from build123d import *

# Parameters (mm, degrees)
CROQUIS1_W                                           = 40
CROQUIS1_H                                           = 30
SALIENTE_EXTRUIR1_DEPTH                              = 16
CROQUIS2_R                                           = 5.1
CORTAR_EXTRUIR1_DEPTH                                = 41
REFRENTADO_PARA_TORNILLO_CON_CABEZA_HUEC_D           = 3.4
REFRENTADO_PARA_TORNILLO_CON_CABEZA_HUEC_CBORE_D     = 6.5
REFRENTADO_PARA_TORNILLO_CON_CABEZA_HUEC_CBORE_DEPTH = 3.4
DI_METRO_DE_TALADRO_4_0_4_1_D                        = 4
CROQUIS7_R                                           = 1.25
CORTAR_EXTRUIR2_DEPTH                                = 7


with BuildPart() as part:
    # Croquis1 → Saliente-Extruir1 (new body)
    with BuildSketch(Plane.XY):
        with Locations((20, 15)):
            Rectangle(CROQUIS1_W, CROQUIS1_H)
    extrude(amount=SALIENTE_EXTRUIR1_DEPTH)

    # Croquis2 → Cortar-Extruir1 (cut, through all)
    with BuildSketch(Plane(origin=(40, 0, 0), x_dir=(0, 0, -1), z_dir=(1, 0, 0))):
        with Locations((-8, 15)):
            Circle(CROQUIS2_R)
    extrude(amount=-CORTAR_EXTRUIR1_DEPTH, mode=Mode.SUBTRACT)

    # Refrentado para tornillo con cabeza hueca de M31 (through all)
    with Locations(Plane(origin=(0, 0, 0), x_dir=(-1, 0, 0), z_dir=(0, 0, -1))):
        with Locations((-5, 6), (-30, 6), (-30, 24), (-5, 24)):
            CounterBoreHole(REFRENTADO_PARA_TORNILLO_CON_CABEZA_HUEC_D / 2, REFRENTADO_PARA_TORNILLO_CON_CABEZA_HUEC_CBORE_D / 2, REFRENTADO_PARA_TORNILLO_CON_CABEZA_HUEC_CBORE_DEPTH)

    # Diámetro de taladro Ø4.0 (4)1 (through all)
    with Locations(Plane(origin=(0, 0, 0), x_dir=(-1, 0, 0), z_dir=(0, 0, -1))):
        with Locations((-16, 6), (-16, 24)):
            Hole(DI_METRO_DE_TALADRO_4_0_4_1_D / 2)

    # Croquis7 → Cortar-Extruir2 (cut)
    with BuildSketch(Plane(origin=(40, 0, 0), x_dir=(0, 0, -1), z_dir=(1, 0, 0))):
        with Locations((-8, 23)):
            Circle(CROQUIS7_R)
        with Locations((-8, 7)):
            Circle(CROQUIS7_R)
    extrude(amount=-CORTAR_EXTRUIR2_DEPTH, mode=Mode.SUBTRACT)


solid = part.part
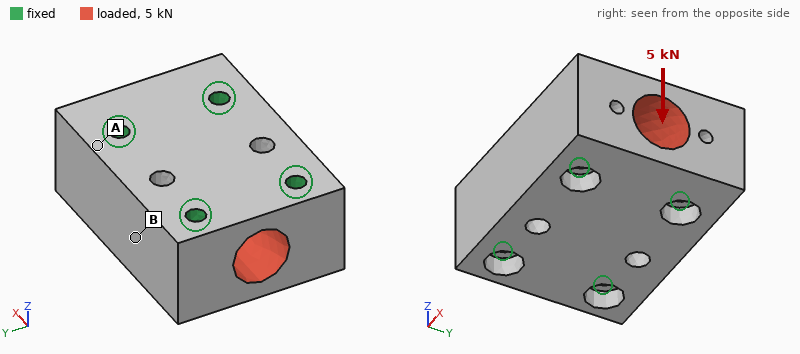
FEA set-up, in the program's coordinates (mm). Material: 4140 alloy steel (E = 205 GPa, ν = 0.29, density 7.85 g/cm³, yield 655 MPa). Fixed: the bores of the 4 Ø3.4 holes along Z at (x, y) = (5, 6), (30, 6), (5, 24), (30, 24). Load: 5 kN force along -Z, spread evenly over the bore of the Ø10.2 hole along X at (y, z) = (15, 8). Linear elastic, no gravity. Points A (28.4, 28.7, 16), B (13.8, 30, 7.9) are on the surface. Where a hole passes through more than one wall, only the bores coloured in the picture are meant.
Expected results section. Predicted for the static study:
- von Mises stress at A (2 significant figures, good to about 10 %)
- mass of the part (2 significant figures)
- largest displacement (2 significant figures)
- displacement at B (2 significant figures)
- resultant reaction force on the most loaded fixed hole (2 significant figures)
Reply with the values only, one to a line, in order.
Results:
6.4 MPa
110 g
1.2 µm
0.27 µm
1.4 kN
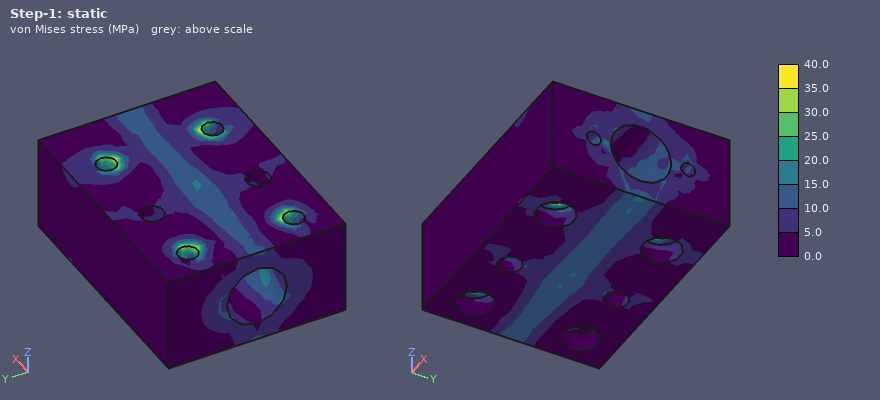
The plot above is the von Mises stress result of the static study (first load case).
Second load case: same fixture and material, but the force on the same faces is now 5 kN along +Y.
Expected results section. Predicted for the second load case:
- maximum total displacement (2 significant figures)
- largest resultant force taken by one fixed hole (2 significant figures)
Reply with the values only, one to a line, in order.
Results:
0.72 µm
1.4 kN
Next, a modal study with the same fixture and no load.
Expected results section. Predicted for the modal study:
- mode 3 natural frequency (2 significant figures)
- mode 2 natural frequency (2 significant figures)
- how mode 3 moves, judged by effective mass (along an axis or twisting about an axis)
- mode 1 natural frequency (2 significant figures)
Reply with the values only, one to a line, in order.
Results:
50 kHz
48 kHz
along Z
46 kHz
